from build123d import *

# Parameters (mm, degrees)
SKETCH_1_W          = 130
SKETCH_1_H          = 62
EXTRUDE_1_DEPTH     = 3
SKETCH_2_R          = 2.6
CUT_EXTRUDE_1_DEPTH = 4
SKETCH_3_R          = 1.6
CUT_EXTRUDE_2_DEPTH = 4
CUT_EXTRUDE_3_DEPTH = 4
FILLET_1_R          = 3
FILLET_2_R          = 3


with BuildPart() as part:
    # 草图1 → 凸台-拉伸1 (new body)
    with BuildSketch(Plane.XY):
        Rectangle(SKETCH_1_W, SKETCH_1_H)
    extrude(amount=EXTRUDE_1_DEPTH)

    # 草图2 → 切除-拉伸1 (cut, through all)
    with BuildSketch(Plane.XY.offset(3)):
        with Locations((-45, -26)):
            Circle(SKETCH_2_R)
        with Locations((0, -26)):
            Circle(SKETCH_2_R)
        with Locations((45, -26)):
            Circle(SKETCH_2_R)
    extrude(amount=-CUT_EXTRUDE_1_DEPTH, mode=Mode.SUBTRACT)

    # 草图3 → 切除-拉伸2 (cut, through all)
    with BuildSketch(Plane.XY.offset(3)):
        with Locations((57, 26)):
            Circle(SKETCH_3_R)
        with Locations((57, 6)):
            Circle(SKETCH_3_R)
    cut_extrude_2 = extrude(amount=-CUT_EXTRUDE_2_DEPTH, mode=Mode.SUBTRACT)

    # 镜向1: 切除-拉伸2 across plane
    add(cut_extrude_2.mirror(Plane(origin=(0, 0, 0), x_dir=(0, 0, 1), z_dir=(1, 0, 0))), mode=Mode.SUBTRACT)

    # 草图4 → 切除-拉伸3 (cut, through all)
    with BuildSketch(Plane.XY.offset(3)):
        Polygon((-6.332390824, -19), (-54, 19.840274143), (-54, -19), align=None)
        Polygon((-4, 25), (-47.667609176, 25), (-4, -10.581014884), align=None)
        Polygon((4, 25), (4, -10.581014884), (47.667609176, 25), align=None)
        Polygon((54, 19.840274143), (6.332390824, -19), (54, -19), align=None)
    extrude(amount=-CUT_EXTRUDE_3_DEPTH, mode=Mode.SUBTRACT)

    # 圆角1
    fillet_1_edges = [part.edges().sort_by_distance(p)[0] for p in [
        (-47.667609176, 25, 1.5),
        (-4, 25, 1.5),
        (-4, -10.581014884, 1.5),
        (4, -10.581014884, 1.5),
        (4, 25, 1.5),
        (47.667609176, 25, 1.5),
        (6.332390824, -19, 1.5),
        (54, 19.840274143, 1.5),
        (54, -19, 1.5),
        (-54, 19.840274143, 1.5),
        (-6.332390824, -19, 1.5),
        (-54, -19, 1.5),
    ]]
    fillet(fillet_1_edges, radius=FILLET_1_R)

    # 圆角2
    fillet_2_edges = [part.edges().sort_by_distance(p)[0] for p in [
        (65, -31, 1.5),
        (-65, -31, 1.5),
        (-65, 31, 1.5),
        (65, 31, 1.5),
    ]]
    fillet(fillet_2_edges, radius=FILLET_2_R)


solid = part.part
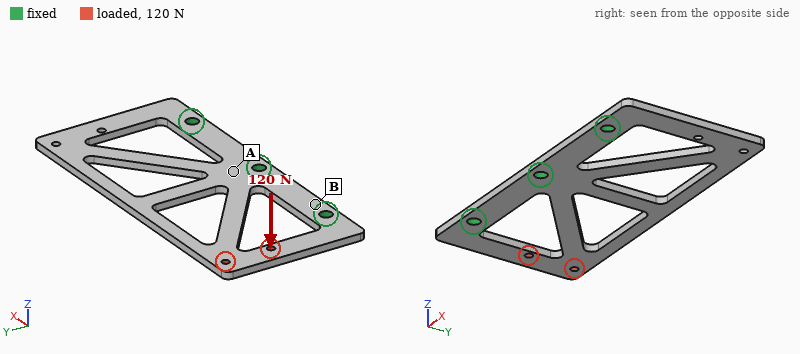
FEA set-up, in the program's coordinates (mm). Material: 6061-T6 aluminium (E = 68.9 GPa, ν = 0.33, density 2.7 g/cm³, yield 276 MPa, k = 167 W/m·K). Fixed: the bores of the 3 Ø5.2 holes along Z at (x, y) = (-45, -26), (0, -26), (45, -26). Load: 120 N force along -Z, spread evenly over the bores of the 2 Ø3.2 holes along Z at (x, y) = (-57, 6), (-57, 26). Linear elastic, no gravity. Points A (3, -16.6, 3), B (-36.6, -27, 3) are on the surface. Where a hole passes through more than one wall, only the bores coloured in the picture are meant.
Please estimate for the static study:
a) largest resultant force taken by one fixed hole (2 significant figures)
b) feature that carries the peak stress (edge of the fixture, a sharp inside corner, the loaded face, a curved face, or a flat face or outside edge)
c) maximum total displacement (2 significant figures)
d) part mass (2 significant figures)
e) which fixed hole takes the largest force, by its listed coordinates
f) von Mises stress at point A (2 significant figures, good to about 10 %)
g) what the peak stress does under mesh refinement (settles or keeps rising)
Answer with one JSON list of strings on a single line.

["96 N", "edge of the fixture", "1.6 mm", "38 g", "(-45, -26)", "42 MPa", "keeps rising"]
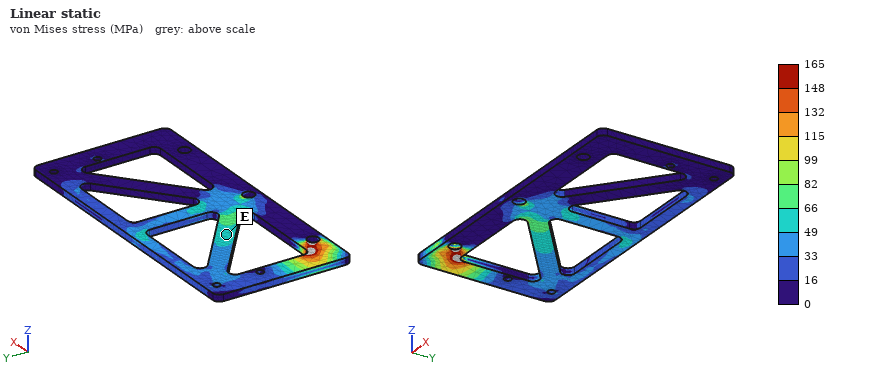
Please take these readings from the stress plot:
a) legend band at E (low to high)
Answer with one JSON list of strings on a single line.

["49 to 66 MPa"]
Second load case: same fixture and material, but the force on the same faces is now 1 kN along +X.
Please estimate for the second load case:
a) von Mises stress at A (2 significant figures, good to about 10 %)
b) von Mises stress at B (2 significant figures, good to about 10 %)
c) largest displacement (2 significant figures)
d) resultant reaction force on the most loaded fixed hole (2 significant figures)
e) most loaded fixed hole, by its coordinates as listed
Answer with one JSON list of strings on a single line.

["19 MPa", "9.6 MPa", "86 µm", "620 N", "(0, -26)"]
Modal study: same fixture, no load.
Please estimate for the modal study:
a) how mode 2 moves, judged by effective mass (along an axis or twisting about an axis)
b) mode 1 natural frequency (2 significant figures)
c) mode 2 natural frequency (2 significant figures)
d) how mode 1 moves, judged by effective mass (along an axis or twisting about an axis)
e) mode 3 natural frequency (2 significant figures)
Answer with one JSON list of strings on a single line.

["twisting about Y", "540 Hz", "700 Hz", "along Z", "1400 Hz"]
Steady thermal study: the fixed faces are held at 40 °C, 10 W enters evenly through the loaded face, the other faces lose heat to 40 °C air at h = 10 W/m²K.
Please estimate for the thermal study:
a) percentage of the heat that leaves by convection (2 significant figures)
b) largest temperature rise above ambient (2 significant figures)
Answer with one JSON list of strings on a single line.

["12 %", "42 K"]
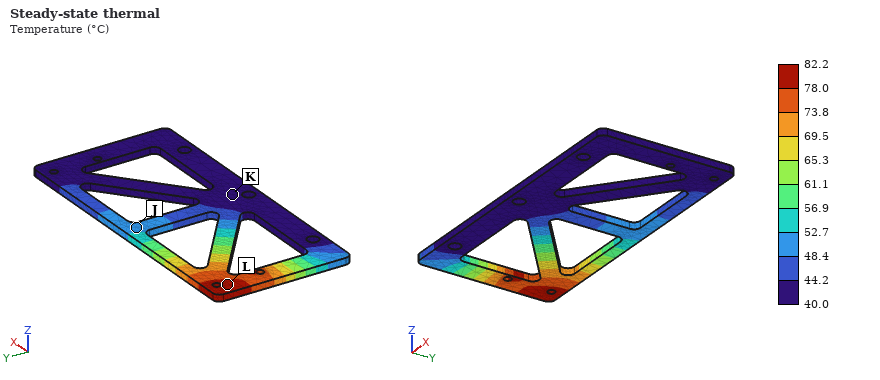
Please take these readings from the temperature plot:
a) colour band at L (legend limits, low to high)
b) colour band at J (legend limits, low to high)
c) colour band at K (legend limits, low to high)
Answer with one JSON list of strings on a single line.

["78.0 to 82.2 °C", "48.4 to 52.7 °C", "40.0 to 44.2 °C"]
